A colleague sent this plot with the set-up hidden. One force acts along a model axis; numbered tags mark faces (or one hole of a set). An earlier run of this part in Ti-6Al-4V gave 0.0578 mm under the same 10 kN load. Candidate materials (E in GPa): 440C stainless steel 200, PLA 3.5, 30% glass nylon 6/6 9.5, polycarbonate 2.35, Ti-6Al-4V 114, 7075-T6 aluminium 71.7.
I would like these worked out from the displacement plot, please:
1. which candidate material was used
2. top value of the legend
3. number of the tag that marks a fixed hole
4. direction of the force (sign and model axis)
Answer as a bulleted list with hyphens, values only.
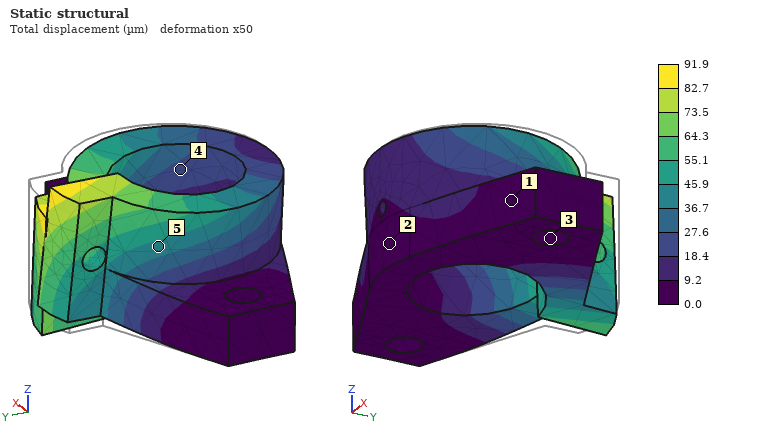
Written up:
- 7075-T6 aluminium
- 91.9 µm
- 3
- -X
